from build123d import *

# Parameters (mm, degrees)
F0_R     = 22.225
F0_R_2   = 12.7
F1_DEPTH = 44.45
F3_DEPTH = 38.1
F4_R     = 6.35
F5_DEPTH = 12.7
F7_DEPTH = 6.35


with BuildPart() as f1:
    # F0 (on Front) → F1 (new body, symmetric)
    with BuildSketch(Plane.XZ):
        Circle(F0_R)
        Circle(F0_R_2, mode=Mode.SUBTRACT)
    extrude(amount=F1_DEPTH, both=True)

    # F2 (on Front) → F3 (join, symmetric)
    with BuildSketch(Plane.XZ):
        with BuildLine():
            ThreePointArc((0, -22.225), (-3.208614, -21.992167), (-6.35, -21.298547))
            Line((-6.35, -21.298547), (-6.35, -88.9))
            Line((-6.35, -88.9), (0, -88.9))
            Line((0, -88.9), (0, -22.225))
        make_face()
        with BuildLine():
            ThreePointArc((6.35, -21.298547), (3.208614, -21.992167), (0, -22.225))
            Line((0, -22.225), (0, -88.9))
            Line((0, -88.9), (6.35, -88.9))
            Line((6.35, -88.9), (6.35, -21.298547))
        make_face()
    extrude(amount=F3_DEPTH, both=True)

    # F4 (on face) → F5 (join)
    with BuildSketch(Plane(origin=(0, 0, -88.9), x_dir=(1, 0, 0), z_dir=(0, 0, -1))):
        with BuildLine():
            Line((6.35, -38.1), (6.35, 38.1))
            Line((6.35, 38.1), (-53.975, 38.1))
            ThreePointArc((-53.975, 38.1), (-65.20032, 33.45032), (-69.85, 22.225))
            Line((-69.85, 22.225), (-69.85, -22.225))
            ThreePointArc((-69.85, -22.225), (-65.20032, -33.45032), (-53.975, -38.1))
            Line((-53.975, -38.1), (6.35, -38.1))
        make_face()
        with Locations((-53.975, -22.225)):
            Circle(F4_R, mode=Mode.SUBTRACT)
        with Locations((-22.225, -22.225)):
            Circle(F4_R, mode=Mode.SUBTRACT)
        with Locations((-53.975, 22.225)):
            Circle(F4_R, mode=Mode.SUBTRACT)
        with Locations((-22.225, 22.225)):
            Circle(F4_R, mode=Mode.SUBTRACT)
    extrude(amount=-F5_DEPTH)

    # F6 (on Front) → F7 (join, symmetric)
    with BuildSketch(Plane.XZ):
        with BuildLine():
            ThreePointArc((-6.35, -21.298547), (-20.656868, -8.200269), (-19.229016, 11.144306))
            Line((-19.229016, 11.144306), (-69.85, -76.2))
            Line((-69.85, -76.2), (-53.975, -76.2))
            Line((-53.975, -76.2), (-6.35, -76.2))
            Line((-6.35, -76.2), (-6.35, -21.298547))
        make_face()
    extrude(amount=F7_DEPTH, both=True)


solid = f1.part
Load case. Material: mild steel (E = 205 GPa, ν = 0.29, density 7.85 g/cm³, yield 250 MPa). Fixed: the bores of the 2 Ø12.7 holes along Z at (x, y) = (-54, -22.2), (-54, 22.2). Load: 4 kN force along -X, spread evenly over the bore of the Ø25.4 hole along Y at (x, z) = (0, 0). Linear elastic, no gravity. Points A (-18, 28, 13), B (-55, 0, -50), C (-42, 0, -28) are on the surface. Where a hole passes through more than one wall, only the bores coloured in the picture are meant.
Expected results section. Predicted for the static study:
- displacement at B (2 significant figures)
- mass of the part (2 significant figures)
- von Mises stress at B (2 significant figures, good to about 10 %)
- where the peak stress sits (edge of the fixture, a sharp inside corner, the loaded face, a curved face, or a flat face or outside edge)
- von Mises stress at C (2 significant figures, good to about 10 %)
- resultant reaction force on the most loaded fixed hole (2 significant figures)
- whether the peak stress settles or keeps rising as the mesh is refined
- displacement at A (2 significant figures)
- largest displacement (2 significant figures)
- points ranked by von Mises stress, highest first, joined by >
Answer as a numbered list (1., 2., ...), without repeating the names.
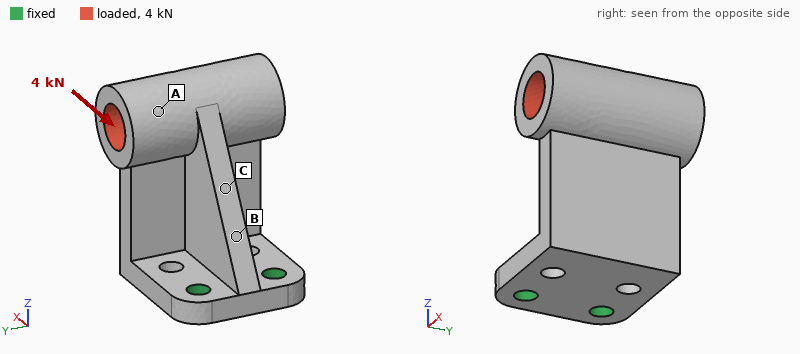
1. 0.039 mm
2. 2.0 kg
3. 44 MPa
4. edge of the fixture
5. 24 MPa
6. 2.0 kN
7. keeps rising
8. 0.13 mm
9. 0.16 mm
10. B > C > A
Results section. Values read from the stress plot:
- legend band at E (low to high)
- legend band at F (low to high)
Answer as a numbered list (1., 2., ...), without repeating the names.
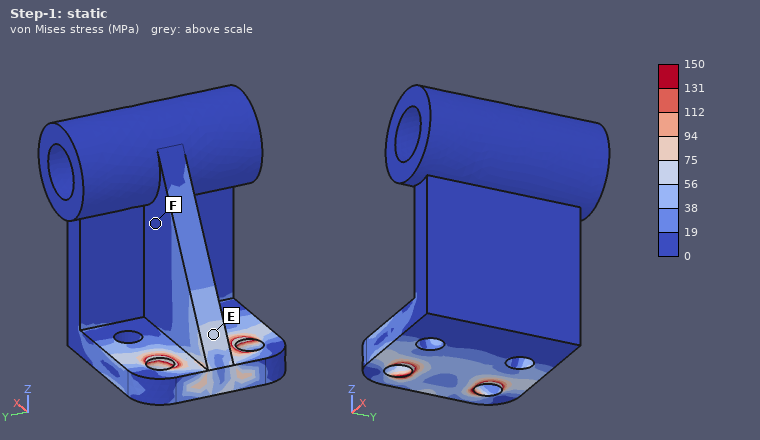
1. 56 to 75 MPa
2. 0 to 19 MPa
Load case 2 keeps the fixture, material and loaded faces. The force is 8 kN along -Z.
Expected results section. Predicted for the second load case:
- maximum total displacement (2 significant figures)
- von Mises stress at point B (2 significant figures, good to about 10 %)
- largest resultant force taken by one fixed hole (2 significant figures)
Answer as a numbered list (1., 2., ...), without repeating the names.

1. 0.18 mm
2. 31 MPa
3. 4.1 kN
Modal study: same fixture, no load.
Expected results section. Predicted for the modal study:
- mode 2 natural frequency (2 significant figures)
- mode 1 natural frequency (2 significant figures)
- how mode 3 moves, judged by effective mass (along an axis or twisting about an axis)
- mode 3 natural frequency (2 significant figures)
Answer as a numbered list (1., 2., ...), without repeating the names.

1. 850 Hz
2. 830 Hz
3. twisting about Z
4. 2300 Hz
